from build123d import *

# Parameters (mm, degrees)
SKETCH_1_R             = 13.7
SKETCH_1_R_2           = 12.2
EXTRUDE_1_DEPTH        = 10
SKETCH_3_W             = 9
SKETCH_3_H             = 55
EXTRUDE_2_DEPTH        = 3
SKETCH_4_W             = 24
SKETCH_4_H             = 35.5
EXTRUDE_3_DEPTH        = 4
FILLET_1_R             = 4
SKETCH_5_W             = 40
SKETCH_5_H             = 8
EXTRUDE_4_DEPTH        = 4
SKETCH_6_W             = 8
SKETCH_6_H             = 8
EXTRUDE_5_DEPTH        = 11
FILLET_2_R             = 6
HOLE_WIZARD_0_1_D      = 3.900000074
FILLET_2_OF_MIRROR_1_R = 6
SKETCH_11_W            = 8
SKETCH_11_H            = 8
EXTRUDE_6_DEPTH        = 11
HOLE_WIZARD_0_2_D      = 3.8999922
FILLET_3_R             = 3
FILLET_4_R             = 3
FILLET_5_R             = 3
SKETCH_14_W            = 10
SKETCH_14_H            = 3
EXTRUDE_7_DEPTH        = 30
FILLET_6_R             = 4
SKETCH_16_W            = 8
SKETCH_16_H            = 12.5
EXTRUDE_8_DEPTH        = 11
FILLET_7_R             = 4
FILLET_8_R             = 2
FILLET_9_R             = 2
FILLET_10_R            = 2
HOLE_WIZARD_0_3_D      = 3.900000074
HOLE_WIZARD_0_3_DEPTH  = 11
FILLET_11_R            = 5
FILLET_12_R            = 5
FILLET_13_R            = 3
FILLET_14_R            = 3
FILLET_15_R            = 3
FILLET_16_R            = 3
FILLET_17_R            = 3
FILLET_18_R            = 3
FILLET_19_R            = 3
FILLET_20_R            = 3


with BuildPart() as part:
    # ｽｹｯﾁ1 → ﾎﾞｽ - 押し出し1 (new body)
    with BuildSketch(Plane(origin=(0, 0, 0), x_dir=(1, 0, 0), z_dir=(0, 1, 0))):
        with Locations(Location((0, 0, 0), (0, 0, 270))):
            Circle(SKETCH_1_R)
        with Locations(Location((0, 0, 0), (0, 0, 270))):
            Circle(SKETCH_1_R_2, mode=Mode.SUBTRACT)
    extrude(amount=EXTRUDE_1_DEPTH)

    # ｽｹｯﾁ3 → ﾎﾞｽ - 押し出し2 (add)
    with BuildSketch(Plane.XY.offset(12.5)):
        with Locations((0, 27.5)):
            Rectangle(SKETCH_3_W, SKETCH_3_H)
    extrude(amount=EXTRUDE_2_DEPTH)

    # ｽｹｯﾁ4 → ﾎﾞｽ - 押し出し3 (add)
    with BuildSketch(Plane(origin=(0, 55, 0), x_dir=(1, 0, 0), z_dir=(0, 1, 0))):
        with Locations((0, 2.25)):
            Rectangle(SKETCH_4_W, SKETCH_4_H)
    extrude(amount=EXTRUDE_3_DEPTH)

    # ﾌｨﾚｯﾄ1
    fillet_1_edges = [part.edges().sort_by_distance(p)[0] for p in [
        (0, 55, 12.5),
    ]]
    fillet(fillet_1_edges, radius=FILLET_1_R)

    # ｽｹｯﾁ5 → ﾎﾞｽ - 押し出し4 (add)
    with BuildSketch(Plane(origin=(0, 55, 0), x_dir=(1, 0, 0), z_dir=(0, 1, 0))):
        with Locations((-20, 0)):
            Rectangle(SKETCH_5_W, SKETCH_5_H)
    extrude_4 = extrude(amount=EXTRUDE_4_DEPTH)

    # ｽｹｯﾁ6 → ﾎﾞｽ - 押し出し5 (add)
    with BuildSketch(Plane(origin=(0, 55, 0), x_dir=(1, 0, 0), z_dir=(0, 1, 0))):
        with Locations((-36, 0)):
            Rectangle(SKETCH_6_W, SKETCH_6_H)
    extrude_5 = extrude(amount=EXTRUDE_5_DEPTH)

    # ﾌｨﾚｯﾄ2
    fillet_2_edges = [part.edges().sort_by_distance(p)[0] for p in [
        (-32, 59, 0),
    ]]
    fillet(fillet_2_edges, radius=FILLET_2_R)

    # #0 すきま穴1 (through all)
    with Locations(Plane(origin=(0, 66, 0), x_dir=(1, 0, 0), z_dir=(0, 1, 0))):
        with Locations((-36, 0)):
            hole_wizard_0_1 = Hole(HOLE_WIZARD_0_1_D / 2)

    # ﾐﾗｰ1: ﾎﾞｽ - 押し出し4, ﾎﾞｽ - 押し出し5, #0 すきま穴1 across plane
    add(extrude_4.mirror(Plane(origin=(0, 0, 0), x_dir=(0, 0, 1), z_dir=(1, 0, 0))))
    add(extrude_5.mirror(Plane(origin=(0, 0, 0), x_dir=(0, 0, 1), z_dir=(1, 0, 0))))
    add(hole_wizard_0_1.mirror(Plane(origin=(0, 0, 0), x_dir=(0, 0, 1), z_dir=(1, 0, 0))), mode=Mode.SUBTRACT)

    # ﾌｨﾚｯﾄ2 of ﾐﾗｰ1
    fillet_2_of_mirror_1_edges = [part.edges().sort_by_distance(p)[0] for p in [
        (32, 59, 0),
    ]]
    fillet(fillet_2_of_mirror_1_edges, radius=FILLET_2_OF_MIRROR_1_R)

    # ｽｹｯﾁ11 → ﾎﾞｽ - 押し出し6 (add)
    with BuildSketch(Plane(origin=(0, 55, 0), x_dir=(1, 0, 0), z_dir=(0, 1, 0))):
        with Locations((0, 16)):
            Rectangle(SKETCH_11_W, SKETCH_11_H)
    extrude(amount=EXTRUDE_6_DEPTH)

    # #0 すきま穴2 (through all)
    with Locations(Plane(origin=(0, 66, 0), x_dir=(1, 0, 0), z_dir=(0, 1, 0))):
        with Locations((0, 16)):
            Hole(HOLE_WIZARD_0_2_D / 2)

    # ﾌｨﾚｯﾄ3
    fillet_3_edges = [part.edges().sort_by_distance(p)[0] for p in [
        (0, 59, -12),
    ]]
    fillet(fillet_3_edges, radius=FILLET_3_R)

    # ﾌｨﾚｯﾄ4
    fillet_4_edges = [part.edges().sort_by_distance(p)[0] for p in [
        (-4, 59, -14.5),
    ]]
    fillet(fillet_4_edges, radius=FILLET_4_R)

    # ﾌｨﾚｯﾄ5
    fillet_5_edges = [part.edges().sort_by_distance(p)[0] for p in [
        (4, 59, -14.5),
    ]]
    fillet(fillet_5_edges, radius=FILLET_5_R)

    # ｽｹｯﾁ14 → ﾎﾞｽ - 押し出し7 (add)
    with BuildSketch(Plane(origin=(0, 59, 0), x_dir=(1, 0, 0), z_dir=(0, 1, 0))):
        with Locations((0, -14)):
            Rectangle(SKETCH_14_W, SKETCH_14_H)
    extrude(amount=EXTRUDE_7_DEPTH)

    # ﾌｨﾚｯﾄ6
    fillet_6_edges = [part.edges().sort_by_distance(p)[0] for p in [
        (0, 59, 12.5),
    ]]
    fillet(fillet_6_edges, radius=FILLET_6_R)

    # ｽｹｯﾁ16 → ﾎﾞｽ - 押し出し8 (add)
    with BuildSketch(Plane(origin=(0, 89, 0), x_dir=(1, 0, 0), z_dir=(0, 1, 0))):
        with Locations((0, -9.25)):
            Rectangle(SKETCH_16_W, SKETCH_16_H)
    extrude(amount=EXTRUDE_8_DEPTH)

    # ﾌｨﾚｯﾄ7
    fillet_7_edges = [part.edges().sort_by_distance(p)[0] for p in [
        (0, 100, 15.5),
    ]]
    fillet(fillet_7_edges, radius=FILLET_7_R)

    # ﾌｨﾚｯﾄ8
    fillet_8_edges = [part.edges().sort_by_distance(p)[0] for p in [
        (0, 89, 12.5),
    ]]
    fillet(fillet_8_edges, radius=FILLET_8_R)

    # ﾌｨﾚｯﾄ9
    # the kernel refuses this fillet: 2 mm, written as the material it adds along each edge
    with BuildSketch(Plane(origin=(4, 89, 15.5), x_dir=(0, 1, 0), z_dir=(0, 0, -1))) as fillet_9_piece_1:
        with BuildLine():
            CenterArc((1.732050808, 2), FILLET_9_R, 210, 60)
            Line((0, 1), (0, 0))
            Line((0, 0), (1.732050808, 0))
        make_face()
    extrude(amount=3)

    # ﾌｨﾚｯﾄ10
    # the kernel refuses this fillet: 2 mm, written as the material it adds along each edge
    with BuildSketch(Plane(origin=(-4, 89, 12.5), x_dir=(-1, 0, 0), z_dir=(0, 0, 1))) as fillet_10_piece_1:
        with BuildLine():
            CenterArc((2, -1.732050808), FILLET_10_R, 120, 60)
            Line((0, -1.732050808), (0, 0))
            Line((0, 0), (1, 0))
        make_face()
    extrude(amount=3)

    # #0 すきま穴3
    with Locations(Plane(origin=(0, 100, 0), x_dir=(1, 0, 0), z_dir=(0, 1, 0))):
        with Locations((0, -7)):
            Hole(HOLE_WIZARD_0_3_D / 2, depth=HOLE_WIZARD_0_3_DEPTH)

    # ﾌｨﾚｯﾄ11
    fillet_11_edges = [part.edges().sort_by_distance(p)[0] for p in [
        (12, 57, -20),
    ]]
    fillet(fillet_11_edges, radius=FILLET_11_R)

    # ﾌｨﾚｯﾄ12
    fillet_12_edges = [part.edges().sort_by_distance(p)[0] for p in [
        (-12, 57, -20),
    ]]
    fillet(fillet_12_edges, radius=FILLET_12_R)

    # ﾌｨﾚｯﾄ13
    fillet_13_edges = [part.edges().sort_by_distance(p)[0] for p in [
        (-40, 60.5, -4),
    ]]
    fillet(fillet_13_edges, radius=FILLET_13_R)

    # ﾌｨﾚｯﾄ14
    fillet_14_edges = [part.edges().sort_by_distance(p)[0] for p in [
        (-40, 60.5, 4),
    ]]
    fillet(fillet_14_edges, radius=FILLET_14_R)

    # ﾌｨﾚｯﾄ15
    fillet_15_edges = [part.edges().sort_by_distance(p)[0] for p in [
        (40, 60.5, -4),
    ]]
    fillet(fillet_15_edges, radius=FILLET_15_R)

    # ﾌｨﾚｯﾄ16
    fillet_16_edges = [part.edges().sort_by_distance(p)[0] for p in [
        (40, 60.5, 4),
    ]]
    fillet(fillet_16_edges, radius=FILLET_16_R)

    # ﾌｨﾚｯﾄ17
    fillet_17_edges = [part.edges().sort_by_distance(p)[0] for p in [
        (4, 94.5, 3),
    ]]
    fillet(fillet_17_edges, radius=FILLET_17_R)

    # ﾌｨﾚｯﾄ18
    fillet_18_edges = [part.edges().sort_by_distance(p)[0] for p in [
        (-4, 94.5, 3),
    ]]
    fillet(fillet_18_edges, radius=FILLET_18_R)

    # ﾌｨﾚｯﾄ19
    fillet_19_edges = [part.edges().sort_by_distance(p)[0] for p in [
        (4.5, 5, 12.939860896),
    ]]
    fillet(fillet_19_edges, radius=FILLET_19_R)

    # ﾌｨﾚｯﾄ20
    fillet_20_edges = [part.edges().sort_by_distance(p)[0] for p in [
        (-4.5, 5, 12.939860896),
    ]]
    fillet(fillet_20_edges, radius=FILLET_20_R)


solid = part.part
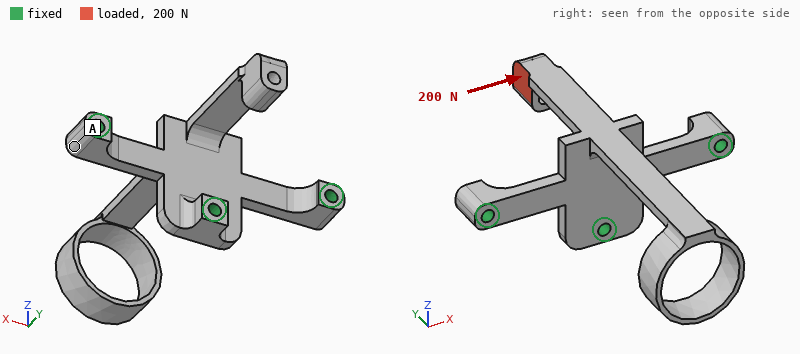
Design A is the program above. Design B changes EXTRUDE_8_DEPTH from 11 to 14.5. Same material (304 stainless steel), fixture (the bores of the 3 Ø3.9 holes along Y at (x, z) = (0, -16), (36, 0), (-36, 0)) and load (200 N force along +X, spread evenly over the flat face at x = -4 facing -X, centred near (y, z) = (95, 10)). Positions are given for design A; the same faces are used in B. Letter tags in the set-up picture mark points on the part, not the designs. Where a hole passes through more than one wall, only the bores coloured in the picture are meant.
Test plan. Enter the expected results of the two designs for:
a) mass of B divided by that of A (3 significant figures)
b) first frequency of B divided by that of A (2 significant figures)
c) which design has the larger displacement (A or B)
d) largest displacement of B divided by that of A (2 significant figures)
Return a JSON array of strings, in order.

["1.03", "1.00", "B", "1.1"]
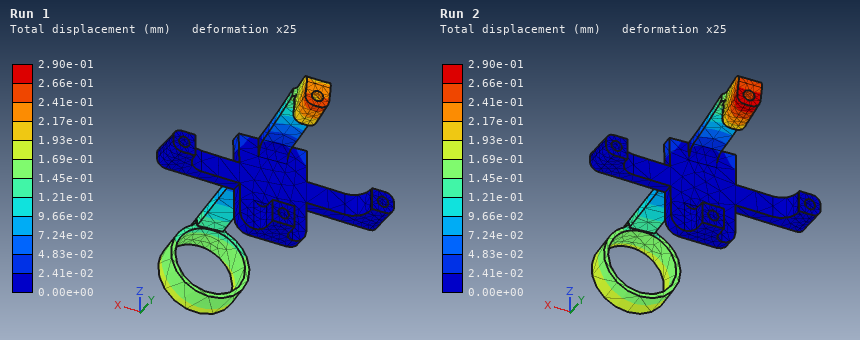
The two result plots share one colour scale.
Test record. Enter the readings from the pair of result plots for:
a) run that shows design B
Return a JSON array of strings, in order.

["Run 2"]
